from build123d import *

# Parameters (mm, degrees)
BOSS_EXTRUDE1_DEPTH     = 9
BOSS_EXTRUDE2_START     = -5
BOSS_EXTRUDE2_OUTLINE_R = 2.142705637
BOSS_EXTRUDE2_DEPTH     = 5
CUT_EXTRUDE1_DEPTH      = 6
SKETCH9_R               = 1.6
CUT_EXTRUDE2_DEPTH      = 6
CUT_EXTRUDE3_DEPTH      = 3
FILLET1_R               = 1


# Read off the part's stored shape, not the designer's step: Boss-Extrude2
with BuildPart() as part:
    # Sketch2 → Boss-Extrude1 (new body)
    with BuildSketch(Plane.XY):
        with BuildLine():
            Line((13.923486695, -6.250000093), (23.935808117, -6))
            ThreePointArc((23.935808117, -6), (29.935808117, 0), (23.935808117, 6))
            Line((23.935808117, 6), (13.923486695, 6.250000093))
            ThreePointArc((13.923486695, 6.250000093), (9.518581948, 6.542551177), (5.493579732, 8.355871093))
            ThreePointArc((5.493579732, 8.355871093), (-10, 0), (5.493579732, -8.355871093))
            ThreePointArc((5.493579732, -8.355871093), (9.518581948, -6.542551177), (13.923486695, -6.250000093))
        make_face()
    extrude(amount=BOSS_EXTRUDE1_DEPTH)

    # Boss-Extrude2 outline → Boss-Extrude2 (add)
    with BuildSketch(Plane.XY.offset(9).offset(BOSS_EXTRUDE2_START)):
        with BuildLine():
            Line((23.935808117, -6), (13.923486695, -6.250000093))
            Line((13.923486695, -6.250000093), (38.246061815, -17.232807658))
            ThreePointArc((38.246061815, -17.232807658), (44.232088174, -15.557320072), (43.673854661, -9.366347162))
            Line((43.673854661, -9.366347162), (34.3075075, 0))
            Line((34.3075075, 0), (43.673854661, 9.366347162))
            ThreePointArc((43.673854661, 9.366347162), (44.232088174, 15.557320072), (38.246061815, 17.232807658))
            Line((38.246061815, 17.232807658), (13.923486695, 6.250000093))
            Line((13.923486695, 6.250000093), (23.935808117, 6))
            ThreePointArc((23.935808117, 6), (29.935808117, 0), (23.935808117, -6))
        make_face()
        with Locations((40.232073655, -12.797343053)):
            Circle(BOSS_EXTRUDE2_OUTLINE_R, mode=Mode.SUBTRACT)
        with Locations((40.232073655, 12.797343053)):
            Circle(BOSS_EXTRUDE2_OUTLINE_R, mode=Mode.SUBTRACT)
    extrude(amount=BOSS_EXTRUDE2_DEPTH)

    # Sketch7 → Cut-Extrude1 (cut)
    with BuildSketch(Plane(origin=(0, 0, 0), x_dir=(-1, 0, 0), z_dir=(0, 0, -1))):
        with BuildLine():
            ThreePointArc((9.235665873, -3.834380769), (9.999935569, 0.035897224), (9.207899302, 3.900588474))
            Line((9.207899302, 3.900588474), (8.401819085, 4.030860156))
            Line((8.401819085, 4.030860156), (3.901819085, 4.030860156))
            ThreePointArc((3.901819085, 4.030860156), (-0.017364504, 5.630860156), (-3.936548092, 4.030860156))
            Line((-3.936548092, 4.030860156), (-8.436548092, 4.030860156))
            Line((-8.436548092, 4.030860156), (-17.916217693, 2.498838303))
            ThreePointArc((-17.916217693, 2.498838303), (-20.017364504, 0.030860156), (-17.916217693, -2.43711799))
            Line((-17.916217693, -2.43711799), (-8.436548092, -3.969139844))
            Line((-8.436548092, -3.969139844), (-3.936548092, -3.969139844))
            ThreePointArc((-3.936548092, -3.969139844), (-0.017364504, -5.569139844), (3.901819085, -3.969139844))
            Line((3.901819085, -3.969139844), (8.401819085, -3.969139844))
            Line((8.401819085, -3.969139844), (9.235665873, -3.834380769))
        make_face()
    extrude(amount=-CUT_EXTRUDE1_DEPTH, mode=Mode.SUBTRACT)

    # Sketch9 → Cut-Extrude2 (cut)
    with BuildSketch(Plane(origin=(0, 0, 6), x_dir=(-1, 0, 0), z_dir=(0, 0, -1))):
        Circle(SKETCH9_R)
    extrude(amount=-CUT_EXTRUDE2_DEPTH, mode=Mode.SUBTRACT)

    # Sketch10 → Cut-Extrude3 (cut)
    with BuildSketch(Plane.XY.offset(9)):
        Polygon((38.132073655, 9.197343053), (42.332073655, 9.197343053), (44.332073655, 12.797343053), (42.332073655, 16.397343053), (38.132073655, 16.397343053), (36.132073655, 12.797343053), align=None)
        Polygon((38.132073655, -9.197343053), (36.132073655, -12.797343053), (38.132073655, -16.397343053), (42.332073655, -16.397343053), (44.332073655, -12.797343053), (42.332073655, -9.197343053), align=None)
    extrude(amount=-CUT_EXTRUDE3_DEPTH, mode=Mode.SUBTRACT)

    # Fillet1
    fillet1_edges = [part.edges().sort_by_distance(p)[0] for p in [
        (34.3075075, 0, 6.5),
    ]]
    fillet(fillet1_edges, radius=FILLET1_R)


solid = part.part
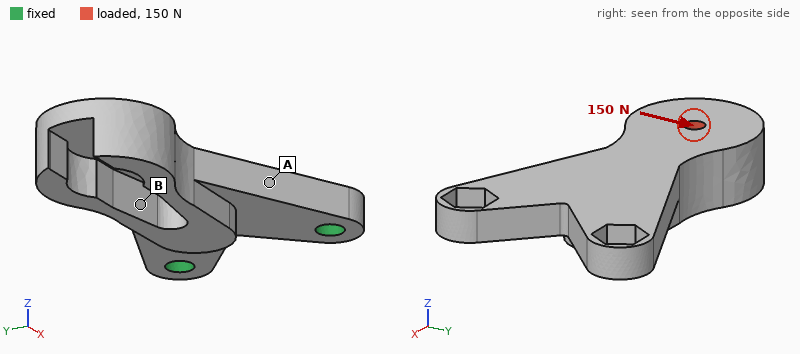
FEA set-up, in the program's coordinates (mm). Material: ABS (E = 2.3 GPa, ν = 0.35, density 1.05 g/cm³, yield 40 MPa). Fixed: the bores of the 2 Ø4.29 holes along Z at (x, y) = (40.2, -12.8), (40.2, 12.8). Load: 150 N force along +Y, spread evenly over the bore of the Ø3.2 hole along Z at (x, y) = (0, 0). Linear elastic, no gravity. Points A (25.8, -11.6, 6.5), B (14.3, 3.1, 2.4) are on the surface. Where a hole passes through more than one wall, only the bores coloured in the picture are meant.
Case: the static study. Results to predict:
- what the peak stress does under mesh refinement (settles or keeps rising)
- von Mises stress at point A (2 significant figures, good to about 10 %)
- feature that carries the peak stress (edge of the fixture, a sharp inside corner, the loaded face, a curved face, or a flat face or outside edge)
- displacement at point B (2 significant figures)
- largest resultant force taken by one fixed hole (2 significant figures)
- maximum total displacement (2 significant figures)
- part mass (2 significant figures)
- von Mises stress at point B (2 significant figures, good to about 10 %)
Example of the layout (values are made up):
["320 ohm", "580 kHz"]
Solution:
["keeps rising", "9.4 MPa", "edge of the fixture", "0.17 mm", "240 N", "0.73 mm", "6.1 g", "3.5 MPa"]
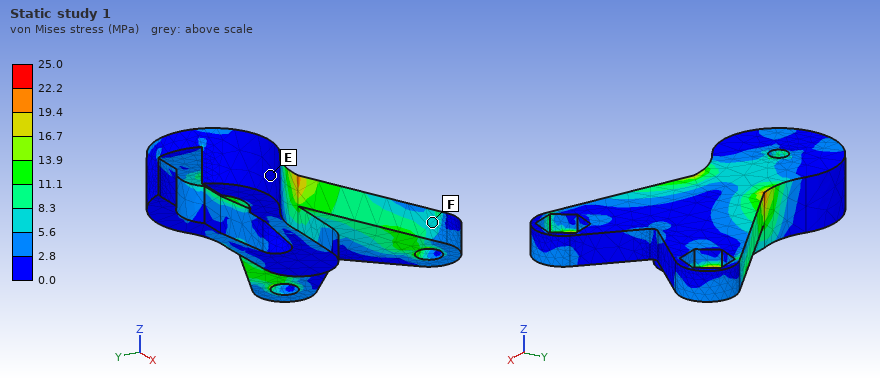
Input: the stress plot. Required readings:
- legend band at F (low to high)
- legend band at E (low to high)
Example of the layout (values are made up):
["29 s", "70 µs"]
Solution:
["5.6 to 8.3 MPa", "0.0 to 2.8 MPa"]
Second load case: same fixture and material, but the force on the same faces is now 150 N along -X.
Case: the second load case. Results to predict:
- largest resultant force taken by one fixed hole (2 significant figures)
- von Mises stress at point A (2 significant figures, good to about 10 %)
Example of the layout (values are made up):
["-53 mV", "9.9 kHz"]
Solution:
["81 N", "1.8 MPa"]
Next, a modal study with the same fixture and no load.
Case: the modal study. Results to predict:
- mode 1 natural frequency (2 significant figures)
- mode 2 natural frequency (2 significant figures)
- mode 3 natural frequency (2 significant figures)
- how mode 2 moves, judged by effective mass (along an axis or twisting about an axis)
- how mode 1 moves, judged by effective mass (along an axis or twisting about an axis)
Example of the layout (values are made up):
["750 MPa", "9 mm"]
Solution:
["400 Hz", "1700 Hz", "2700 Hz", "along Y", "along Z"]
